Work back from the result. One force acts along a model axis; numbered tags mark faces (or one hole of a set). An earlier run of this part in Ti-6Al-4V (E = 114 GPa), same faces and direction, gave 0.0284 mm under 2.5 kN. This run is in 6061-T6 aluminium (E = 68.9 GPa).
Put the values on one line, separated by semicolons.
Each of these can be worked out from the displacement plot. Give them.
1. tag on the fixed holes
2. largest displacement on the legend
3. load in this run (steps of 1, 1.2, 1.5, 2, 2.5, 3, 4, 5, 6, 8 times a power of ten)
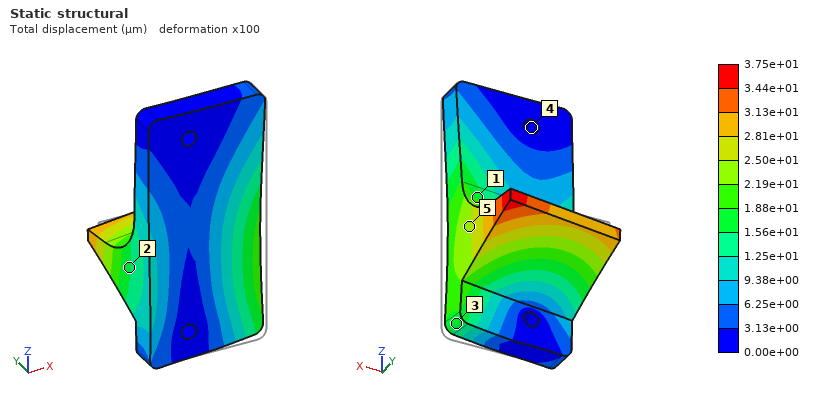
4; 3.75e+01 µm; 2 kN
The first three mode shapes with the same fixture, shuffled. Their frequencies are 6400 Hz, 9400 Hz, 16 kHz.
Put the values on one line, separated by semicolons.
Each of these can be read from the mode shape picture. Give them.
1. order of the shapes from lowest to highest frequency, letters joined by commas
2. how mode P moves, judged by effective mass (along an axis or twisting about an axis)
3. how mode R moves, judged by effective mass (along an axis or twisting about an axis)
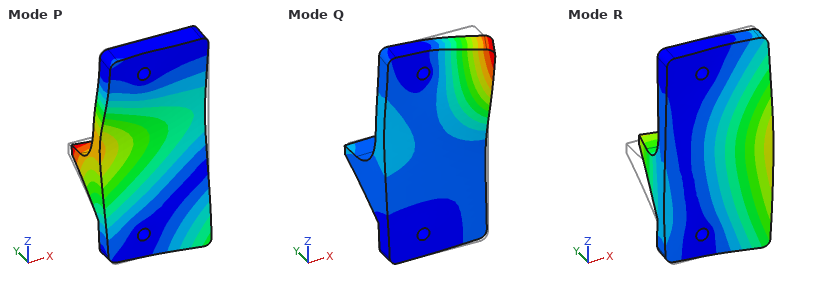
R, P, Q; along Y; along Y
